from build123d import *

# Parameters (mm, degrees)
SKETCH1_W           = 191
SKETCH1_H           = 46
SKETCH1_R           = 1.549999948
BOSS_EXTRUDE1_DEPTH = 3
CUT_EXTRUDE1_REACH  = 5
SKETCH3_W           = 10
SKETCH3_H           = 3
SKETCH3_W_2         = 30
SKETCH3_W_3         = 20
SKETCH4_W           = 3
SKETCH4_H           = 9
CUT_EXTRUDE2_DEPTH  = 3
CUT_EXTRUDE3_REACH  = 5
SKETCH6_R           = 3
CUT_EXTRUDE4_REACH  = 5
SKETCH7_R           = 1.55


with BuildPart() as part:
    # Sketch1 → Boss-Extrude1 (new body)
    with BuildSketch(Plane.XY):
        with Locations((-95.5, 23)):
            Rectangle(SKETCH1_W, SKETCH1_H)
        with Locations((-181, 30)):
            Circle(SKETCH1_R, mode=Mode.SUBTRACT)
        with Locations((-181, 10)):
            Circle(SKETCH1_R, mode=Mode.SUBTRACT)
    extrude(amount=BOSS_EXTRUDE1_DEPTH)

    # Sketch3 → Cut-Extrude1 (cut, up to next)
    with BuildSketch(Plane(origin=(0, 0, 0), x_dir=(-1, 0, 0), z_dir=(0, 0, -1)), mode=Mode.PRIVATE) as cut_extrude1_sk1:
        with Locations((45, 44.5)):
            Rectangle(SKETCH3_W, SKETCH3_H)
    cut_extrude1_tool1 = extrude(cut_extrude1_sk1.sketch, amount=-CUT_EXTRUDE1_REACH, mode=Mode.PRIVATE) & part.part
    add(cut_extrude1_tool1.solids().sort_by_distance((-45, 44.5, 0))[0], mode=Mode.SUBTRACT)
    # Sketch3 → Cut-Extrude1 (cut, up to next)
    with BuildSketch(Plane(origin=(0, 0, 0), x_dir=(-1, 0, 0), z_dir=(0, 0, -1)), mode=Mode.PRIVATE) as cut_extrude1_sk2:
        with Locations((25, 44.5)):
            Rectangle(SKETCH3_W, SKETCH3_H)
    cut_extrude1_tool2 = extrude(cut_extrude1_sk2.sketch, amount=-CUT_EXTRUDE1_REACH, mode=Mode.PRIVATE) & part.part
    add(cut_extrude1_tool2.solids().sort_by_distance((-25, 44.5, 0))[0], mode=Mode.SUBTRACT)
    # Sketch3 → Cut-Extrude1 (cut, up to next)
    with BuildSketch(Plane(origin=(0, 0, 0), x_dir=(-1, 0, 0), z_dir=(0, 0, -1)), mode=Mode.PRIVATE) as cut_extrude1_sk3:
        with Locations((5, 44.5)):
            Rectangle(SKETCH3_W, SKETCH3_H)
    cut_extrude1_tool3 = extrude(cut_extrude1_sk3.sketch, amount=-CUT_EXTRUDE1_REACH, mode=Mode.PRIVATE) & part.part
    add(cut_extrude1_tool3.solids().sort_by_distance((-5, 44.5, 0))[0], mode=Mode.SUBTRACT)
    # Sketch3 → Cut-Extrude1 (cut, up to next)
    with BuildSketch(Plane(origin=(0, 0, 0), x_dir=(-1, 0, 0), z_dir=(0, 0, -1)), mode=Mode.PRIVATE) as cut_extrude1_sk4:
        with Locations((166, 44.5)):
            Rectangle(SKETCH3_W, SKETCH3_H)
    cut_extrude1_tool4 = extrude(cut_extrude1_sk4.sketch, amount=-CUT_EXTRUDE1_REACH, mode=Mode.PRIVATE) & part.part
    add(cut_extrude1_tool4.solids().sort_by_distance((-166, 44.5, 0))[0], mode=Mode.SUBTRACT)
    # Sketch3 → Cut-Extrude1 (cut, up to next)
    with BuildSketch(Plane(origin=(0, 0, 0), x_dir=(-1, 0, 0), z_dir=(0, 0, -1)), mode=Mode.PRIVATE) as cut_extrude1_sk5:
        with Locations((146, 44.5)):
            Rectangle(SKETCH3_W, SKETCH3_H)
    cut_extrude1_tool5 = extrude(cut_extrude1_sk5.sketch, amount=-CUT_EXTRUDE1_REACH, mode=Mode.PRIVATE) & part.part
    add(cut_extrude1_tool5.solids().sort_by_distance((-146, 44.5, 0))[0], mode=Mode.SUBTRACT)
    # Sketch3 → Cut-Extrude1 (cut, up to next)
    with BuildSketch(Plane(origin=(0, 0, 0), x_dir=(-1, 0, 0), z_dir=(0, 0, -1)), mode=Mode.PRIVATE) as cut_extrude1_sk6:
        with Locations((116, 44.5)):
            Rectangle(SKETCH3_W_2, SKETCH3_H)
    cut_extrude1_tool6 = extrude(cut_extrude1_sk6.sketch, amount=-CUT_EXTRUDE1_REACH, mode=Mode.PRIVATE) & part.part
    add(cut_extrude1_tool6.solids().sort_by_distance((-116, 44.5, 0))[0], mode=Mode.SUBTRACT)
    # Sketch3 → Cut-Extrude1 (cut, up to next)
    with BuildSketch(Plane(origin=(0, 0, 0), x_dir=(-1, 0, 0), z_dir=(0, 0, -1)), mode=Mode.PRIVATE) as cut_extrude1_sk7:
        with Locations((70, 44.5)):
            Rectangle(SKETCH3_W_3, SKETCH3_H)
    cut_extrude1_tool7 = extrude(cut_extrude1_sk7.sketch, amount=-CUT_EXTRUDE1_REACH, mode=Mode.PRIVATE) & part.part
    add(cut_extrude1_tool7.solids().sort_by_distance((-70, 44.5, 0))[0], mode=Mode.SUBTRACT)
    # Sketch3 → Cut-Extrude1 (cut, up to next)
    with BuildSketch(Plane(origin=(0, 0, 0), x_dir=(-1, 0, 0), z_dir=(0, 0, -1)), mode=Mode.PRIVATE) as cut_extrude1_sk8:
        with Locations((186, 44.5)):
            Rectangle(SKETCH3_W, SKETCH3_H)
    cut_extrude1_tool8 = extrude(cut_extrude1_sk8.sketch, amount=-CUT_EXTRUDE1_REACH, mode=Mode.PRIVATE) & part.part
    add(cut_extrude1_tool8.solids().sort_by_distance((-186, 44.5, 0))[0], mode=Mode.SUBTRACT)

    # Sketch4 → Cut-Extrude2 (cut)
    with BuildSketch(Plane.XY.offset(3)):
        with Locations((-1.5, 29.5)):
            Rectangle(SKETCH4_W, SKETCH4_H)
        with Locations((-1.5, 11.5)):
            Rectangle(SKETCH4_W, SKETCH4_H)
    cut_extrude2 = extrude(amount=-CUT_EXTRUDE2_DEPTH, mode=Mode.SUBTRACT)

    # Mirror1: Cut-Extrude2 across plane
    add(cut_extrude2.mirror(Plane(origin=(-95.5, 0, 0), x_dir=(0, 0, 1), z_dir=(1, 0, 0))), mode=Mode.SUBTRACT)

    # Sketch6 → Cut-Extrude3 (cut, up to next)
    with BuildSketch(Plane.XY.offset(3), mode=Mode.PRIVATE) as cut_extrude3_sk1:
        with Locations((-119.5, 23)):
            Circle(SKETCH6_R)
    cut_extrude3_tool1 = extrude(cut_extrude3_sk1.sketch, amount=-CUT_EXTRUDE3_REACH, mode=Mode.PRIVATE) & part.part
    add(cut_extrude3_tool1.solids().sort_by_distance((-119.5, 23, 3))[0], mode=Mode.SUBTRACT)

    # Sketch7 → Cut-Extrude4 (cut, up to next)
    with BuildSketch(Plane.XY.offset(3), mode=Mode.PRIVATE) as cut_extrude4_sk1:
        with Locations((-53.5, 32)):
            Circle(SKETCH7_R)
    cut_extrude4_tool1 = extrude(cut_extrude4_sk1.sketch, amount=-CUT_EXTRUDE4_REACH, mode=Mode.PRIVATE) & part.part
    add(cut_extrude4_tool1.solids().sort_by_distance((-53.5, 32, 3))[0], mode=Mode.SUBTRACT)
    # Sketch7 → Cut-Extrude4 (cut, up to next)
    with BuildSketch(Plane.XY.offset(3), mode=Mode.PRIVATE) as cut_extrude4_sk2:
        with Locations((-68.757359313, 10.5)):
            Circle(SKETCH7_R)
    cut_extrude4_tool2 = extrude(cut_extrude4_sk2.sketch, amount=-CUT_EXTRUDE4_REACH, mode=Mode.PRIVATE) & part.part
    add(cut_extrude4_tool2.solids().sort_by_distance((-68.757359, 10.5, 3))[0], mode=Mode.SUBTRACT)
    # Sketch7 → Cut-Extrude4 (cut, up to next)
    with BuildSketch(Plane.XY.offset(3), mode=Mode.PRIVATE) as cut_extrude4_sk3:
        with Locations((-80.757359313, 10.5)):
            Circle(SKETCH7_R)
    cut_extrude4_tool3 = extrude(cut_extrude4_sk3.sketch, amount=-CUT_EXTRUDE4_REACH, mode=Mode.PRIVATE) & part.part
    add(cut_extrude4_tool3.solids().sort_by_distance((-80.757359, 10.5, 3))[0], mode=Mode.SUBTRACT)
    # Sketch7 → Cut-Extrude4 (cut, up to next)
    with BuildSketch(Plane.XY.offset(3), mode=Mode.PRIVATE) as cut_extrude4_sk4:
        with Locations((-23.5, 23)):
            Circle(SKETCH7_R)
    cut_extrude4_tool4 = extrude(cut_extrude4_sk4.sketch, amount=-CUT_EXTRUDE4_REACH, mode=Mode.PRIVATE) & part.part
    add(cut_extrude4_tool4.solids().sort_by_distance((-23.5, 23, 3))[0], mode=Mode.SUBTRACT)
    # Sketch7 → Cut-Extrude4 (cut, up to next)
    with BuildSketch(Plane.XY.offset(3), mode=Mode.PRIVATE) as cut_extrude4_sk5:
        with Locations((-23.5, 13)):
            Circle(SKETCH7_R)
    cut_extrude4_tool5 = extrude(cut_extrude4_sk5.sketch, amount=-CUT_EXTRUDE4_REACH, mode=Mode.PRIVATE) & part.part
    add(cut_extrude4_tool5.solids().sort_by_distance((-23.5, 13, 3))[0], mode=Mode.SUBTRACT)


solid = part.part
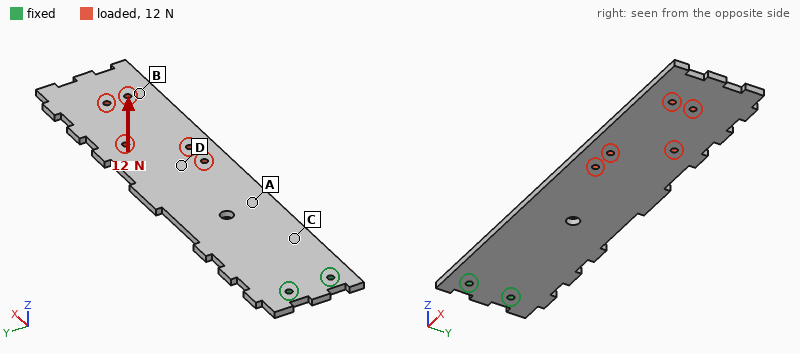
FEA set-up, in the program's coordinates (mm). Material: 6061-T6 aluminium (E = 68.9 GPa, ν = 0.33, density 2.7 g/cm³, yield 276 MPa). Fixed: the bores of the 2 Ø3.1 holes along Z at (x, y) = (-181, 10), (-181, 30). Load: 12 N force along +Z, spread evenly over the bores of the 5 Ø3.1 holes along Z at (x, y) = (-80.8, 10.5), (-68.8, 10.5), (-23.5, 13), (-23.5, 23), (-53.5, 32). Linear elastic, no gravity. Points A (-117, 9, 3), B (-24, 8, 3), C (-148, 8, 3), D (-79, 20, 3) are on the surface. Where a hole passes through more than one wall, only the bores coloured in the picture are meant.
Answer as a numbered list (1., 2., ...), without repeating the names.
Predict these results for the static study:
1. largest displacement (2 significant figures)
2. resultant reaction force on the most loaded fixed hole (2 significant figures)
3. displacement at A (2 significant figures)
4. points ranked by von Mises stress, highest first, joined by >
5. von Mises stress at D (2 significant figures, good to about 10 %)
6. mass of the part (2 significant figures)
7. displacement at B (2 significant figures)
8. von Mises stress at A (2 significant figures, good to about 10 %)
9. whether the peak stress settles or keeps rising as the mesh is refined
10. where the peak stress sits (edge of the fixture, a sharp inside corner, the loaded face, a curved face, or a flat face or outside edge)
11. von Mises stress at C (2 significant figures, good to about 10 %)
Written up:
1. 2.1 mm
2. 6.1 N
3. 0.40 mm
4. C > A > D > B
5. 5.6 MPa
6. 67 g
7. 1.8 mm
8. 13 MPa
9. keeps rising
10. edge of the fixture
11. 18 MPa
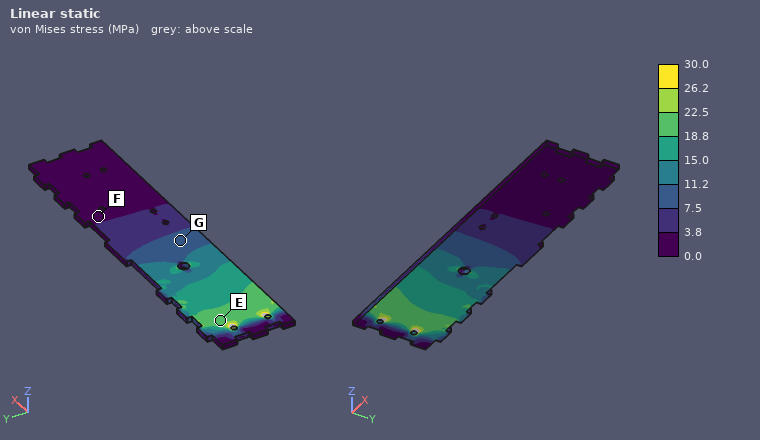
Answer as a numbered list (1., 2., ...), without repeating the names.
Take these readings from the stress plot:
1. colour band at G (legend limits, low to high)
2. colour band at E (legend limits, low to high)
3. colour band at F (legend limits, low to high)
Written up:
1. 7.5 to 11.2 MPa
2. 18.8 to 22.5 MPa
3. 0.0 to 3.8 MPa
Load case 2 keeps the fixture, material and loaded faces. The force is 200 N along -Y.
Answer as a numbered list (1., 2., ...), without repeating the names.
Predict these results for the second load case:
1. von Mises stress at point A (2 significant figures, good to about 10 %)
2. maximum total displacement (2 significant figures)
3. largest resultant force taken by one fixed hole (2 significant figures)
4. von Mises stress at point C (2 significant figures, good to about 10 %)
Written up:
1. 8.6 MPa
2. 0.24 mm
3. 1.2 kN
4. 14 MPa
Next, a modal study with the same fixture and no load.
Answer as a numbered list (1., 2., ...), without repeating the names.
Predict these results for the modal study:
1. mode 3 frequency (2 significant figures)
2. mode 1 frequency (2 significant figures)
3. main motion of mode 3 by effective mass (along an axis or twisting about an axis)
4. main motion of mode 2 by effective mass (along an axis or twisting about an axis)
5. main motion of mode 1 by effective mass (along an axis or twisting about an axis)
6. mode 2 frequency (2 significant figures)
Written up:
1. 590 Hz
2. 75 Hz
3. twisting about X
4. along Z
5. along Z
6. 470 Hz
